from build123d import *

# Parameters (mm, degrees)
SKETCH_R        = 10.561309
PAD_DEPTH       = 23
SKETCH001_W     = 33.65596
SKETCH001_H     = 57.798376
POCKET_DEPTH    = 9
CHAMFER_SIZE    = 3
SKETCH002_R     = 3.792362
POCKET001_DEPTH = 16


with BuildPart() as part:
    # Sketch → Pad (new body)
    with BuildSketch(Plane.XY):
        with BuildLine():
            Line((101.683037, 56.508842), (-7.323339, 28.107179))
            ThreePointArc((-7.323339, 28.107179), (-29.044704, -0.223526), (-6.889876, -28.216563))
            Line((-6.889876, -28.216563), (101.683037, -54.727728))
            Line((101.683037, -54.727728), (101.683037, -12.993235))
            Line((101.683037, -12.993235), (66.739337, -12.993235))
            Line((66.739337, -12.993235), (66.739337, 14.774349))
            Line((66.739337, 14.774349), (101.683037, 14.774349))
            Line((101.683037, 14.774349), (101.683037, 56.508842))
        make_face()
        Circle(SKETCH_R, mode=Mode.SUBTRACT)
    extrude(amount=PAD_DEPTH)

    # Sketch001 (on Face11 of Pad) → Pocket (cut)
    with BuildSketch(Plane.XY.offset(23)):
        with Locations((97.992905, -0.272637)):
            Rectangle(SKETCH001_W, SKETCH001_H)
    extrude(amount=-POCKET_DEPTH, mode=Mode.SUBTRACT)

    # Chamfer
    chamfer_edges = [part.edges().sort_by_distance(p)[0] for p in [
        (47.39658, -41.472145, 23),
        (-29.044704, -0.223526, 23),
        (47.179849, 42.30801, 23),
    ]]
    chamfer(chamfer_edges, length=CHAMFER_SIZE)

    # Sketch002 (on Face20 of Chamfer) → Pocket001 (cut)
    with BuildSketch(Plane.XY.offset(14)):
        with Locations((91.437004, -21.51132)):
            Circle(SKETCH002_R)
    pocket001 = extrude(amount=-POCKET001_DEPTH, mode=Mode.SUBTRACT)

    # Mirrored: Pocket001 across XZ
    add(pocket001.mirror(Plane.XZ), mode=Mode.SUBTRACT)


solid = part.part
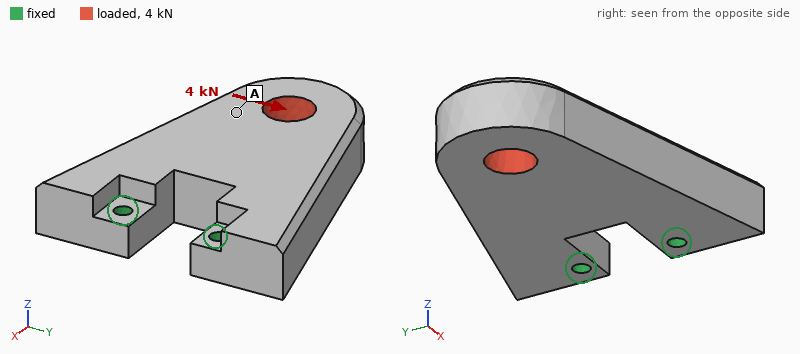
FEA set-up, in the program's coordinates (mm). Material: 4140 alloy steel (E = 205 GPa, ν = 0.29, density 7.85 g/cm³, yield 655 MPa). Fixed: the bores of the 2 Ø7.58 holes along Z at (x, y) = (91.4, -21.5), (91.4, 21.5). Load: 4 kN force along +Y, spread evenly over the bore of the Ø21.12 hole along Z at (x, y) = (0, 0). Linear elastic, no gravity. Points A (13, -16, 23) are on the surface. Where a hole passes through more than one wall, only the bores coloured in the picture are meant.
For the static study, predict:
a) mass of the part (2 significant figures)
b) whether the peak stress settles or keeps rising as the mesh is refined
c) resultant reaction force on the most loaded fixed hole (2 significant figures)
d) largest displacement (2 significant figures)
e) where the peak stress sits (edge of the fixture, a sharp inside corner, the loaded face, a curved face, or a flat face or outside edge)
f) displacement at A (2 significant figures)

1.5 kg
keeps rising
6.5 kN
28 µm
edge of the fixture
18 µm
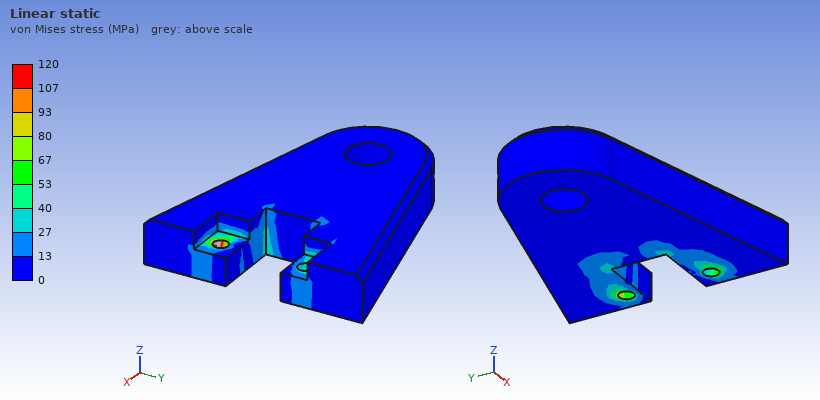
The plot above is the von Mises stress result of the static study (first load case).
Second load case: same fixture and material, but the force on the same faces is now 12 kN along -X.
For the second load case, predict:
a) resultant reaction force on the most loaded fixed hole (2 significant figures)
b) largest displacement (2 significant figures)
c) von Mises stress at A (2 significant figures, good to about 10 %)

6.1 kN
28 µm
10 MPa
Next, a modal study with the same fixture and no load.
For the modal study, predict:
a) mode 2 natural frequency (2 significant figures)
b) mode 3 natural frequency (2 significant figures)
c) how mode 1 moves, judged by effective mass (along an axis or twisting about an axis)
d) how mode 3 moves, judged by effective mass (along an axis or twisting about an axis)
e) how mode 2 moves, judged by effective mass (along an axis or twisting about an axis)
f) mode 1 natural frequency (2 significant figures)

2500 Hz
3700 Hz
along Z
twisting about X
along Y
980 Hz
